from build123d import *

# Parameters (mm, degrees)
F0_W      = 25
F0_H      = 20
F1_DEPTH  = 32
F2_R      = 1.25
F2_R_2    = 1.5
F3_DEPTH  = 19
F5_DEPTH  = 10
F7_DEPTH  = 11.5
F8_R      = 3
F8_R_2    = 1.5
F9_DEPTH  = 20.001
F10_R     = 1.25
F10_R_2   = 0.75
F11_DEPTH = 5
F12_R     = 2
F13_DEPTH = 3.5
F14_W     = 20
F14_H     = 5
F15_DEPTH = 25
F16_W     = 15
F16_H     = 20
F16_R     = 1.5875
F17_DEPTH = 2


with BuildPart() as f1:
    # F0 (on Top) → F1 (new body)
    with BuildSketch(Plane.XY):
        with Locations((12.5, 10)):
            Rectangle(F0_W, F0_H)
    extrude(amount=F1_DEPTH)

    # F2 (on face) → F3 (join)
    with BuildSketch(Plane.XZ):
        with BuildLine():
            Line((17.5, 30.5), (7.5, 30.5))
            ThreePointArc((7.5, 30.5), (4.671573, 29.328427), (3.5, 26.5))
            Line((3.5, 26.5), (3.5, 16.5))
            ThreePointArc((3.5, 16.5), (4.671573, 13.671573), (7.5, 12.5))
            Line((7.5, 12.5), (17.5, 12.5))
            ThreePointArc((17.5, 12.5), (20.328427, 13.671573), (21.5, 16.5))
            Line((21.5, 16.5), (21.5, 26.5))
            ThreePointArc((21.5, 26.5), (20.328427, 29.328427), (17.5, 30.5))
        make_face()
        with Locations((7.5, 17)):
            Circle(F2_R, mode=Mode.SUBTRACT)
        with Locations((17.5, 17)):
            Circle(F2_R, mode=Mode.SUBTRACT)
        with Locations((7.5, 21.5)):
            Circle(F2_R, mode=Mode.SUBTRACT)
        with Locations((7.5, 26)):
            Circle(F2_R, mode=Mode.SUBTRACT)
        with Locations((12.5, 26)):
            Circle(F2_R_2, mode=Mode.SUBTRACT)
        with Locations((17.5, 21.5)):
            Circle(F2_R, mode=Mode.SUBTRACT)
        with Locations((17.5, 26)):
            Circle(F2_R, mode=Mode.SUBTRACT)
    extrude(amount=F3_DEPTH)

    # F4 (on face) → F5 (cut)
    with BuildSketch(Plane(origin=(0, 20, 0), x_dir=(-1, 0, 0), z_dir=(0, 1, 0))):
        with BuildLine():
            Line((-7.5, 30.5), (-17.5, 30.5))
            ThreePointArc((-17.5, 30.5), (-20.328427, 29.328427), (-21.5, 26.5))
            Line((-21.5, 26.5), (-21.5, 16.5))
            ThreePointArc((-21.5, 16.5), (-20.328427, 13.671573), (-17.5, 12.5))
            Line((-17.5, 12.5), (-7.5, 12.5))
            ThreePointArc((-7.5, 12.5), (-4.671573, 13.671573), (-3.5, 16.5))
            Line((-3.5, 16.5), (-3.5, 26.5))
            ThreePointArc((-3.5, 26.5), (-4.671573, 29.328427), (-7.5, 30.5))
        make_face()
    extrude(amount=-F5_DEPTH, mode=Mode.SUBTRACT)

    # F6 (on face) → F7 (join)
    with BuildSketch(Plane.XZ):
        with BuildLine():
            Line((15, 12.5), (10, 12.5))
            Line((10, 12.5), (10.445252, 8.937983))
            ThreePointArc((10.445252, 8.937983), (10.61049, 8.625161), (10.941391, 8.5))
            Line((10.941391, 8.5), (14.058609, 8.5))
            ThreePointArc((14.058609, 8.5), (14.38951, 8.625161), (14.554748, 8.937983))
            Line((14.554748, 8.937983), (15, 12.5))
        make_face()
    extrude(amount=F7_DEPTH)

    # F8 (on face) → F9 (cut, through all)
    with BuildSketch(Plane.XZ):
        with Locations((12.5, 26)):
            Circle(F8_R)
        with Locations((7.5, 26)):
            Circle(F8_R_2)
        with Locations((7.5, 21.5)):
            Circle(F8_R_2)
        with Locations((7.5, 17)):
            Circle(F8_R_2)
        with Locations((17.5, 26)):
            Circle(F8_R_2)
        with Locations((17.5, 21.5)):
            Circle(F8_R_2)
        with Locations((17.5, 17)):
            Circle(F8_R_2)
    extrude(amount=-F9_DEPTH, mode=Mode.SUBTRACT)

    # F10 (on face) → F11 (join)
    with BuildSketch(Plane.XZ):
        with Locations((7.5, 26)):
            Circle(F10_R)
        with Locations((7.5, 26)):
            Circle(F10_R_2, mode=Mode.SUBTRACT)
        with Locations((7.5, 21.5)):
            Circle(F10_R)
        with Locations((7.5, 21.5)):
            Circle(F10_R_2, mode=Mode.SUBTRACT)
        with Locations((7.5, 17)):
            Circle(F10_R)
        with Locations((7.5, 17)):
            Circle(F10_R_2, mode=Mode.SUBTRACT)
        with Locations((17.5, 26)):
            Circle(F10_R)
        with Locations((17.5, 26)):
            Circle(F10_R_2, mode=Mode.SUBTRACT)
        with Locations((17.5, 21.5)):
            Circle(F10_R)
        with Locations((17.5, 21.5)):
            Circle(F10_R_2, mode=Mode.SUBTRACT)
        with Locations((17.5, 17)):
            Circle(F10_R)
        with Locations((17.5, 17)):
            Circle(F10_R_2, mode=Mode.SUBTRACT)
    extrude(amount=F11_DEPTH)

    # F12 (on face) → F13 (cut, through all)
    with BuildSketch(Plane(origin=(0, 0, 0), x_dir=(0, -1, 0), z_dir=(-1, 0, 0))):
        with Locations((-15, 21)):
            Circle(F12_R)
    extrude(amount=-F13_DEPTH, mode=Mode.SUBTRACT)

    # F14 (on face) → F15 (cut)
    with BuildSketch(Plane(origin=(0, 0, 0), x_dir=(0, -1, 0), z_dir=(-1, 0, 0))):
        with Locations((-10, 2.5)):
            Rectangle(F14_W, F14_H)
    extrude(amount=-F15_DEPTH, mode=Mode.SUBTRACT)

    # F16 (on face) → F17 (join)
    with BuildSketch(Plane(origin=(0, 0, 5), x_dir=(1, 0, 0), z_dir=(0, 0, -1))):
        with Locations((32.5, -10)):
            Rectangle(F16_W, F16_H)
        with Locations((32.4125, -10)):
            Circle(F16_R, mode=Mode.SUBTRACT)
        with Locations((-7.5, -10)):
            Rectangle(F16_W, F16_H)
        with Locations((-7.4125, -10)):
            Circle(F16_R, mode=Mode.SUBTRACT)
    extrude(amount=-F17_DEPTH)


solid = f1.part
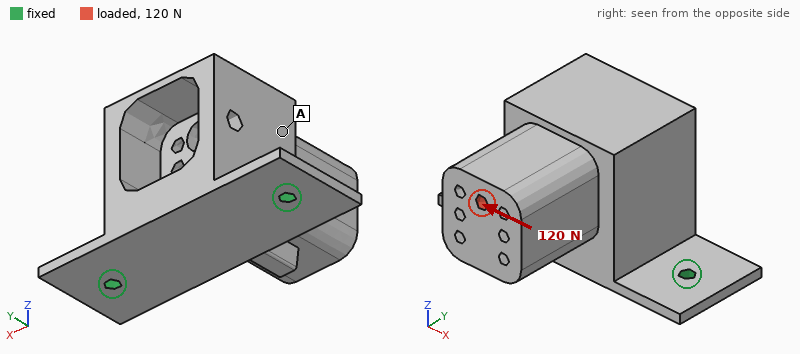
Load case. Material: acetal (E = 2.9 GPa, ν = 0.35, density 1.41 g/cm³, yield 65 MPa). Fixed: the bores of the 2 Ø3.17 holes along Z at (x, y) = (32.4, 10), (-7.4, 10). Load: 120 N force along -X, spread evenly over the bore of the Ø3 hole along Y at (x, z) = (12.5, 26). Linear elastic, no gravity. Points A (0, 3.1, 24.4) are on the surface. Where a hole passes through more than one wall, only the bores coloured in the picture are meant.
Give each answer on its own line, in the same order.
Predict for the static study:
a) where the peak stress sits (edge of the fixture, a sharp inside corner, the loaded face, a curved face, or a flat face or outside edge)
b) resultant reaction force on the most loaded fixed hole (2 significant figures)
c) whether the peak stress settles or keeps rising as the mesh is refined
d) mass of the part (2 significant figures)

edge of the fixture
110 N
keeps rising
23 g
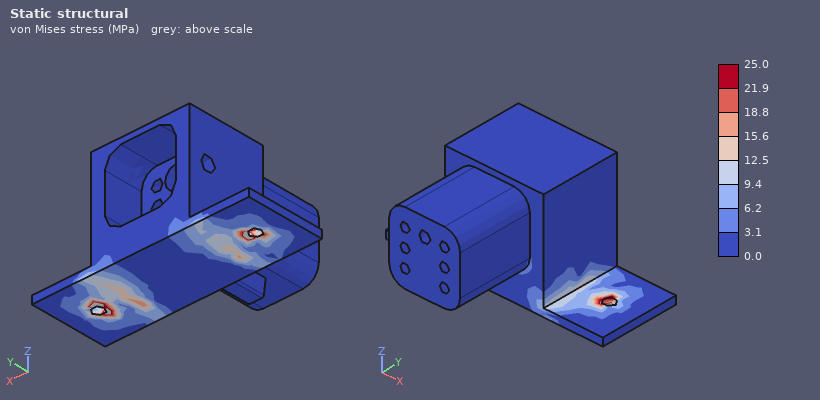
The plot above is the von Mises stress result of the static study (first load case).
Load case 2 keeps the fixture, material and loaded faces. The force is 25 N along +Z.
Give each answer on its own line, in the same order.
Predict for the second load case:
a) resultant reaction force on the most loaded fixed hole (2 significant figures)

14 N
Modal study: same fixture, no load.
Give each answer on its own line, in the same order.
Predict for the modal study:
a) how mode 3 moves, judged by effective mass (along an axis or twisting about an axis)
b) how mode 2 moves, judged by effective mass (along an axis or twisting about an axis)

along Z
along X
